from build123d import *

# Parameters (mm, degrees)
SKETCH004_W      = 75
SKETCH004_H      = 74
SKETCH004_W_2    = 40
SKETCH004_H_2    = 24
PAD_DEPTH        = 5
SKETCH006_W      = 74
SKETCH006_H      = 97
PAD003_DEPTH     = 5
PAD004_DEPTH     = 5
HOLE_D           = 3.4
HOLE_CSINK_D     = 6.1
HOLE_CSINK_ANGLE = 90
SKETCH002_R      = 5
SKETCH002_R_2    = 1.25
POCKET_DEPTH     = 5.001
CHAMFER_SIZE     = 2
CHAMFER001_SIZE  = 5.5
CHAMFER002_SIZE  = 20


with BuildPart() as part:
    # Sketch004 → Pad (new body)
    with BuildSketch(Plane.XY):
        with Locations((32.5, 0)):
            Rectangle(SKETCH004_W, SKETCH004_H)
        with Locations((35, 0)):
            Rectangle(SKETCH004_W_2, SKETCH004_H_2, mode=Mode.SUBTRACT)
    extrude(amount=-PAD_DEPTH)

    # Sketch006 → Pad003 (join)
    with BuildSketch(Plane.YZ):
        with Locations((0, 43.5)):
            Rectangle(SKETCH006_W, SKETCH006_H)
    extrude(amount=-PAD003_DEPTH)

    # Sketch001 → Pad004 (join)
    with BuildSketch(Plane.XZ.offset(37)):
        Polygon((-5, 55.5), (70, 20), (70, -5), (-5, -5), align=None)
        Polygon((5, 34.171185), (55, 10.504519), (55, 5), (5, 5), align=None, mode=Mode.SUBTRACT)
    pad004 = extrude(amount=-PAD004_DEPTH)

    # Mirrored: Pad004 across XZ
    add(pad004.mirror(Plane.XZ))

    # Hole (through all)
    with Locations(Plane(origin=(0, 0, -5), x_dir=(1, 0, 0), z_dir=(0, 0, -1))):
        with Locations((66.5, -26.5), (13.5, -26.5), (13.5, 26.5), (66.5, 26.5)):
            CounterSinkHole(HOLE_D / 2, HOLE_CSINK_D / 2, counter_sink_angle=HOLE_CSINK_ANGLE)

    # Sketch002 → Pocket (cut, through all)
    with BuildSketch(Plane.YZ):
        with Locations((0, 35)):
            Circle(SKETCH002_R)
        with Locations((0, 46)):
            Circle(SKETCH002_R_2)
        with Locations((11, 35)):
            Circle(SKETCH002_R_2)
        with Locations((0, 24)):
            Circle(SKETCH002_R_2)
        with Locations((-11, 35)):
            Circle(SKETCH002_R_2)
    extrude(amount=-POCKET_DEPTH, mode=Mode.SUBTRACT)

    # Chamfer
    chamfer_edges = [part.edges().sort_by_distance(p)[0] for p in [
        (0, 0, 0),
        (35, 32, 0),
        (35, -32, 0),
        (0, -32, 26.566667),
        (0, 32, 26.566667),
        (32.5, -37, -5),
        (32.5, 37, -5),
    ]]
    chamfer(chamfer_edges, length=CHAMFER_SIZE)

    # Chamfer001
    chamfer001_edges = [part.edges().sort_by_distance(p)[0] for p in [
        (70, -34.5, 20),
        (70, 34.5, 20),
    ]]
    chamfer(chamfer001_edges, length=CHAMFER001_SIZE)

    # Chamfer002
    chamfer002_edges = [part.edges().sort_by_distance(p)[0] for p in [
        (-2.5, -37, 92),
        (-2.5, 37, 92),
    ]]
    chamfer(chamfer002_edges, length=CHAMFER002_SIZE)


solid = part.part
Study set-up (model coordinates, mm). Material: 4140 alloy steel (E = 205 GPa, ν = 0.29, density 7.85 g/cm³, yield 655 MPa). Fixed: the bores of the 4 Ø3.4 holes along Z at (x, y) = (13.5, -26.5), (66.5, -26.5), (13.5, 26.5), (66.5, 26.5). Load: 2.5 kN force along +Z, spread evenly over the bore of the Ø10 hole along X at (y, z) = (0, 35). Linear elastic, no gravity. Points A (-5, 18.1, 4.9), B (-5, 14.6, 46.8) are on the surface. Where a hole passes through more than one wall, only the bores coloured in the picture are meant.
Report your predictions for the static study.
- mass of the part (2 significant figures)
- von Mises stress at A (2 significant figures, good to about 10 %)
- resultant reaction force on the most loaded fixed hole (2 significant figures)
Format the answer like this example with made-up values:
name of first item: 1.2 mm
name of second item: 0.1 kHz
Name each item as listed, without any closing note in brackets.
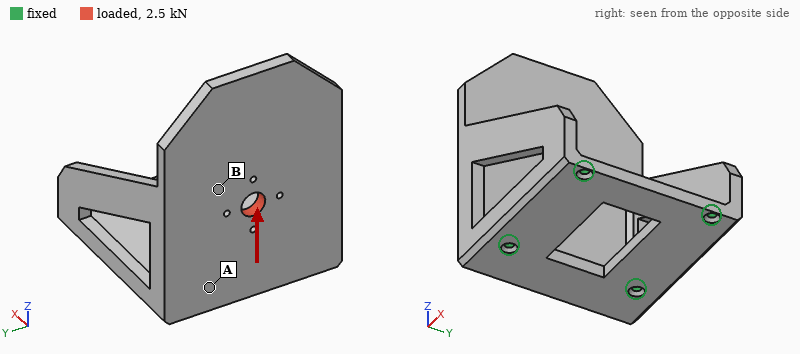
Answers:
mass of the part: 560 g
von Mises stress at A: 17 MPa
resultant reaction force on the most loaded fixed hole: 1.6 kN
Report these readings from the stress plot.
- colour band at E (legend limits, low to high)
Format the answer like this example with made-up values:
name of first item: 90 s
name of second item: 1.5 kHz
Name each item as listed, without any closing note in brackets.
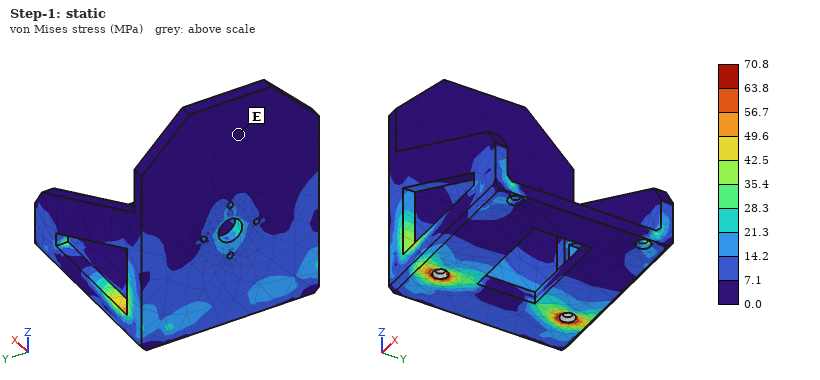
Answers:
colour band at E: 0.0 to 7.1 MPa
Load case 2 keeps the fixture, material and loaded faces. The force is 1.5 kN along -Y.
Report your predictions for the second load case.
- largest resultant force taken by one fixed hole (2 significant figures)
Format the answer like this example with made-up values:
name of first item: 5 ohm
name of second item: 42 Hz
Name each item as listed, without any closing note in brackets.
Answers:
largest resultant force taken by one fixed hole: 1.4 kN
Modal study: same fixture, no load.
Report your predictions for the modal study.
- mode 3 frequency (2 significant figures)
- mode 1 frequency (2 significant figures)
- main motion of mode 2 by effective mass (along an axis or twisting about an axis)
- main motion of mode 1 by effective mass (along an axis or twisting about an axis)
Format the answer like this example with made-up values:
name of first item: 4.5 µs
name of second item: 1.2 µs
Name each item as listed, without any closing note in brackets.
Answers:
mode 3 frequency: 3000 Hz
mode 1 frequency: 1400 Hz
main motion of mode 2 by effective mass: along Y
main motion of mode 1 by effective mass: along X
